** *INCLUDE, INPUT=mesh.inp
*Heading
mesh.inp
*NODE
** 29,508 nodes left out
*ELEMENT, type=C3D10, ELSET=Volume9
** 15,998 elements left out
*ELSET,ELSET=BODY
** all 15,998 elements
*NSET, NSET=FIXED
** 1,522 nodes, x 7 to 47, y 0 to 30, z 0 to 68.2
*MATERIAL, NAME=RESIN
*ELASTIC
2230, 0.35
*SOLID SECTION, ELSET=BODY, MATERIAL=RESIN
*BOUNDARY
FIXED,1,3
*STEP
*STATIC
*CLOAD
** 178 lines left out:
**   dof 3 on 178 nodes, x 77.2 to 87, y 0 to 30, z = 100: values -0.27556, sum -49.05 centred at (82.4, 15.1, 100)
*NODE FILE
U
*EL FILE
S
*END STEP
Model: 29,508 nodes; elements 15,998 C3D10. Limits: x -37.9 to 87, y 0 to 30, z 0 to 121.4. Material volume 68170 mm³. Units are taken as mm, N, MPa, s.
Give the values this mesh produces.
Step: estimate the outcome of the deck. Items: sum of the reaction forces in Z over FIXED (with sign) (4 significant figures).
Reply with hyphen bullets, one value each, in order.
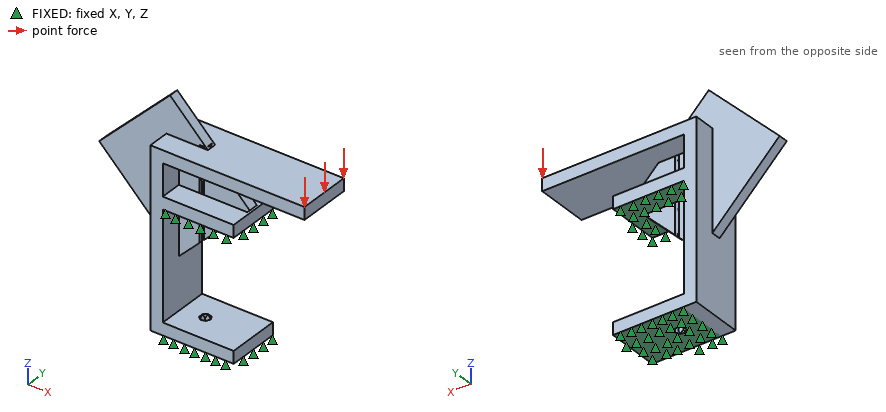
- 49.05 N
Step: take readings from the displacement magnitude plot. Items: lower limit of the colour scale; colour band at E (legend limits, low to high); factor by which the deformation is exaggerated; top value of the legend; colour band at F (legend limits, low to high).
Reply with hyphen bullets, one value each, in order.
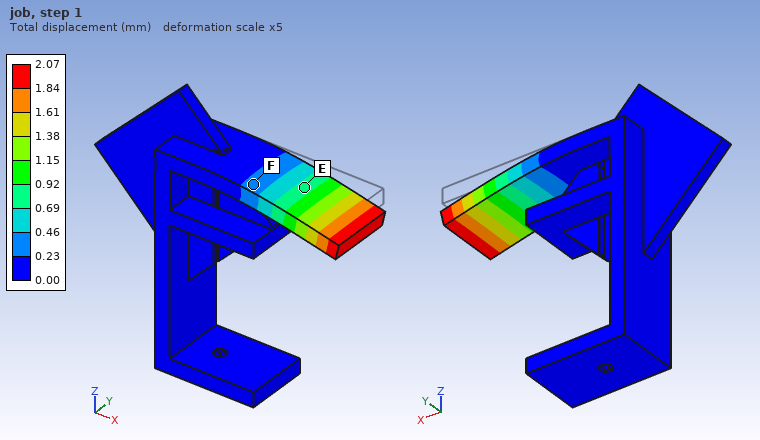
- 0.00 mm
- 0.69 to 0.92 mm
- 5
- 2.07 mm
- 0.23 to 0.46 mm
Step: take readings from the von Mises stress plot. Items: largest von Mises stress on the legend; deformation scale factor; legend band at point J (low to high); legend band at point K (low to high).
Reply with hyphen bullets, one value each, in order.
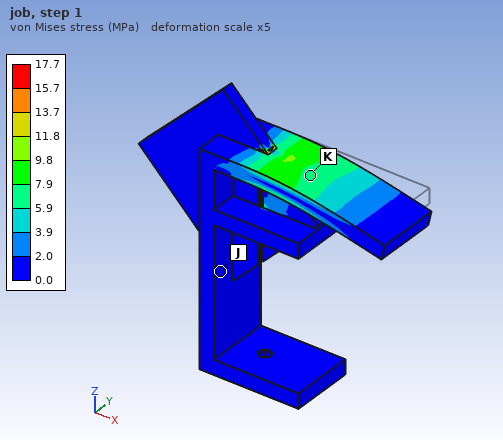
- 17.7 MPa
- 5
- 0.0 to 2.0 MPa
- 5.9 to 7.9 MPa
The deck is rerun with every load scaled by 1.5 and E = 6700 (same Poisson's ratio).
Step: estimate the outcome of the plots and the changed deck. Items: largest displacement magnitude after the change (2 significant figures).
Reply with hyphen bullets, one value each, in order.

- 1.0 mm
